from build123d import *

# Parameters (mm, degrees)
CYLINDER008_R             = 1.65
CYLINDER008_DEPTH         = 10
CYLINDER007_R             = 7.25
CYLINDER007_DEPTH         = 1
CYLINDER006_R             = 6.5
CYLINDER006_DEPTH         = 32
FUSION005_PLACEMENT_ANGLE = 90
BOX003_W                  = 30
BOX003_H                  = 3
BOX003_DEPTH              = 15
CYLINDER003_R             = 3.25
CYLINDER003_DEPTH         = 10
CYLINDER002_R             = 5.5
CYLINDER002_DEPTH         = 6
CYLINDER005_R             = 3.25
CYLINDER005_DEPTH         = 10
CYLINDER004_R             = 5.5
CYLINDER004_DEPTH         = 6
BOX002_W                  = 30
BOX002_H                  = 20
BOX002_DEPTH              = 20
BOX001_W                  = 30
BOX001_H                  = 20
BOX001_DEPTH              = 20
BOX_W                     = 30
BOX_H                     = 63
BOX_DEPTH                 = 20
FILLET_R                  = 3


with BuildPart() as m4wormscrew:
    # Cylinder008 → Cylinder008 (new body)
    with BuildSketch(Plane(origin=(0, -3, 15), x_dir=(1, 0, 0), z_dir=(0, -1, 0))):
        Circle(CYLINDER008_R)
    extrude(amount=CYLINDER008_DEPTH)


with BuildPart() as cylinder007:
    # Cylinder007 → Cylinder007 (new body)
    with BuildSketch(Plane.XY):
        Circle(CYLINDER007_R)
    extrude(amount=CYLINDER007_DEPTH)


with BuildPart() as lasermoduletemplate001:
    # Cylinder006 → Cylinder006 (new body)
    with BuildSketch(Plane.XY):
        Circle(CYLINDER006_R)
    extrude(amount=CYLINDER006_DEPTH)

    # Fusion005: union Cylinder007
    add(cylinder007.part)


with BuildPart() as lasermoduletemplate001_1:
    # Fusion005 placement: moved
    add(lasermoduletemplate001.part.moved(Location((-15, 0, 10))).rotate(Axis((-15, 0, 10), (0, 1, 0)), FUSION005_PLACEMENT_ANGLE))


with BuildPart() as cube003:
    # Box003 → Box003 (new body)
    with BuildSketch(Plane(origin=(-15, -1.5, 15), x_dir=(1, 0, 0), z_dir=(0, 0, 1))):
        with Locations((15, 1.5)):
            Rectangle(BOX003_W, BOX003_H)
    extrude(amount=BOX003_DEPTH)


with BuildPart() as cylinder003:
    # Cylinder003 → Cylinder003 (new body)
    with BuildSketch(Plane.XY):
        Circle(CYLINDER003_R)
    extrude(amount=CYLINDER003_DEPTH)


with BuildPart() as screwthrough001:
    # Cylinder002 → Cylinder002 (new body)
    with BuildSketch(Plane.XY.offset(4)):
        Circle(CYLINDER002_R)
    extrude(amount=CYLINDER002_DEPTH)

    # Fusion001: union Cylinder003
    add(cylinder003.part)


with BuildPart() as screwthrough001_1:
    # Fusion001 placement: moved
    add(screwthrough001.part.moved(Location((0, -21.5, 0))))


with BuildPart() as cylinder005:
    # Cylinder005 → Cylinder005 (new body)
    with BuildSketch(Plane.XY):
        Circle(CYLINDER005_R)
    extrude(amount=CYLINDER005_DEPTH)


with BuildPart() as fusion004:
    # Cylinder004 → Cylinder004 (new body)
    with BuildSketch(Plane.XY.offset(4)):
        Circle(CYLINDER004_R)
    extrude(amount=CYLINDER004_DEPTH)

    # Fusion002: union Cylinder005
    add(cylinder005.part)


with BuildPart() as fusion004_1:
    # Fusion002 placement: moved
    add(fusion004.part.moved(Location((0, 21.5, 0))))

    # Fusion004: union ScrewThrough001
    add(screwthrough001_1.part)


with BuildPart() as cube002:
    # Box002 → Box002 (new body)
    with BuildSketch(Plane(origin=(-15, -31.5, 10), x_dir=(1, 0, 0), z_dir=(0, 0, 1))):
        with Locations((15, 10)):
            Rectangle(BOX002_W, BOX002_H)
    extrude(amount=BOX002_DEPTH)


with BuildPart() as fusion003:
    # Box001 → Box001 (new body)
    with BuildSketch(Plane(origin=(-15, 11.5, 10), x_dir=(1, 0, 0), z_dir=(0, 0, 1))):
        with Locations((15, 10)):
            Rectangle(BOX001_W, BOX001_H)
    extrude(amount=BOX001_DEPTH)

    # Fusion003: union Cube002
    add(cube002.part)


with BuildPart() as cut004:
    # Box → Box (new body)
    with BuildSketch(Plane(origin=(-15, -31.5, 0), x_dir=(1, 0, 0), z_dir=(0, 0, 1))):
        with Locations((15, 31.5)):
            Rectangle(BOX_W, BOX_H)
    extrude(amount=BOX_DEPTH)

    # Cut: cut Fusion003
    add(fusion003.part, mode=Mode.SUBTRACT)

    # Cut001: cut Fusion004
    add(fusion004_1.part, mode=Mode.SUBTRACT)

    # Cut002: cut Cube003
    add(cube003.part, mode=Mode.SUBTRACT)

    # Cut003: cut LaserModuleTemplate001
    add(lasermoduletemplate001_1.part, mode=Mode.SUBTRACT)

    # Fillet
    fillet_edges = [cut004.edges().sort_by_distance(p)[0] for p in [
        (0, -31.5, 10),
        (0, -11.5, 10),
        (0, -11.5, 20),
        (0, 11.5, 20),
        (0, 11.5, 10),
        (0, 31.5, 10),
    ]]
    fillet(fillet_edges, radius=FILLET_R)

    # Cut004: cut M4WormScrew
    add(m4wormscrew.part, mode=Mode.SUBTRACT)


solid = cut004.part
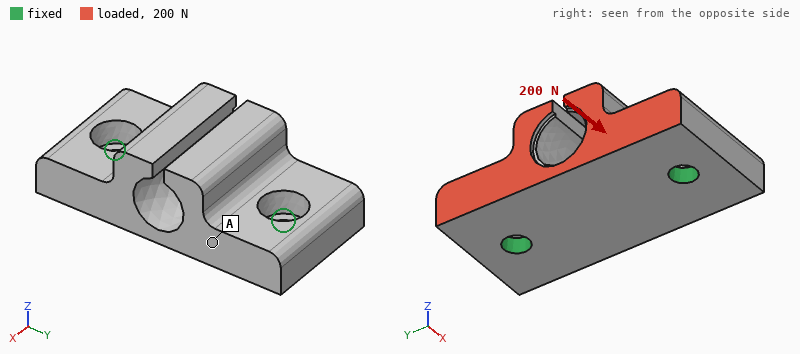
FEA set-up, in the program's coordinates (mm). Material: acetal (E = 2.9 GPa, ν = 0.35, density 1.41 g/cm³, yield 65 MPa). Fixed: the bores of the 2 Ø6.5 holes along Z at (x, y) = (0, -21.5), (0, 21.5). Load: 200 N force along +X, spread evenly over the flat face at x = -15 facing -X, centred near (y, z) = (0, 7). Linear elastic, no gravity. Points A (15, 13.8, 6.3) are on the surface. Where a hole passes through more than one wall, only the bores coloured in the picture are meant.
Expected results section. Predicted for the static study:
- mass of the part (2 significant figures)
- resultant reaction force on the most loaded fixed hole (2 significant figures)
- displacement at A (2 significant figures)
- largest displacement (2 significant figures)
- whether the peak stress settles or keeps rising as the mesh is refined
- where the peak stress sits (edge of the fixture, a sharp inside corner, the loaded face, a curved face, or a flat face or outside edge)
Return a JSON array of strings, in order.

["28 g", "100 N", "28 µm", "48 µm", "keeps rising", "edge of the fixture"]
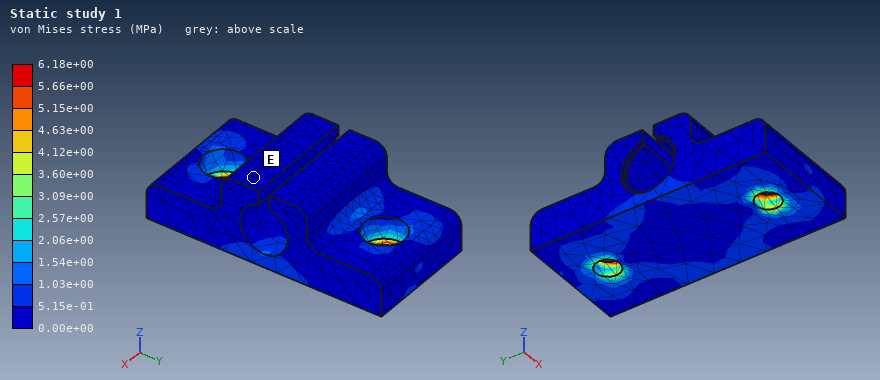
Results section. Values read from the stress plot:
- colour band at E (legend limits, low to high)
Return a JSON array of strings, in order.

["0.00e+00 to 5.15e-01 MPa"]
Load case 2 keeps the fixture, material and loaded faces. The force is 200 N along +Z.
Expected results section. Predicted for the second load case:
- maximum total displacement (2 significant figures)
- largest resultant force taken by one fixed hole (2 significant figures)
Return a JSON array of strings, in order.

["0.16 mm", "100 N"]
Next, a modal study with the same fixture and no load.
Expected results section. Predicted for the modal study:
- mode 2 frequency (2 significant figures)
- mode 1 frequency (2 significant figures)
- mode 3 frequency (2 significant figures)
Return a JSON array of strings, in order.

["2000 Hz", "1900 Hz", "3000 Hz"]
